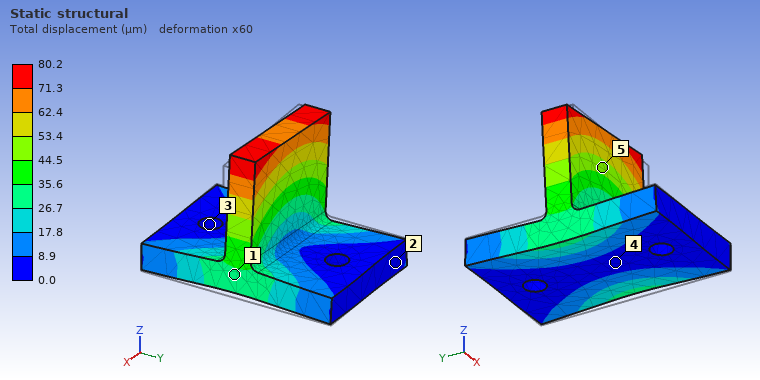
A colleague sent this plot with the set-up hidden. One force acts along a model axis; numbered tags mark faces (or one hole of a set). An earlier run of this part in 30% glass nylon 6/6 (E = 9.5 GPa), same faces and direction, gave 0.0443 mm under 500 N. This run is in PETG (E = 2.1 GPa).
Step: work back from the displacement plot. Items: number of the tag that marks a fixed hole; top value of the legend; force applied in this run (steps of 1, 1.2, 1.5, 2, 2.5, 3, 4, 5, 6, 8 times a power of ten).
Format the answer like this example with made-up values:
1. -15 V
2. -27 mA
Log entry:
1. 3
2. 80.2 µm
3. 200 N
